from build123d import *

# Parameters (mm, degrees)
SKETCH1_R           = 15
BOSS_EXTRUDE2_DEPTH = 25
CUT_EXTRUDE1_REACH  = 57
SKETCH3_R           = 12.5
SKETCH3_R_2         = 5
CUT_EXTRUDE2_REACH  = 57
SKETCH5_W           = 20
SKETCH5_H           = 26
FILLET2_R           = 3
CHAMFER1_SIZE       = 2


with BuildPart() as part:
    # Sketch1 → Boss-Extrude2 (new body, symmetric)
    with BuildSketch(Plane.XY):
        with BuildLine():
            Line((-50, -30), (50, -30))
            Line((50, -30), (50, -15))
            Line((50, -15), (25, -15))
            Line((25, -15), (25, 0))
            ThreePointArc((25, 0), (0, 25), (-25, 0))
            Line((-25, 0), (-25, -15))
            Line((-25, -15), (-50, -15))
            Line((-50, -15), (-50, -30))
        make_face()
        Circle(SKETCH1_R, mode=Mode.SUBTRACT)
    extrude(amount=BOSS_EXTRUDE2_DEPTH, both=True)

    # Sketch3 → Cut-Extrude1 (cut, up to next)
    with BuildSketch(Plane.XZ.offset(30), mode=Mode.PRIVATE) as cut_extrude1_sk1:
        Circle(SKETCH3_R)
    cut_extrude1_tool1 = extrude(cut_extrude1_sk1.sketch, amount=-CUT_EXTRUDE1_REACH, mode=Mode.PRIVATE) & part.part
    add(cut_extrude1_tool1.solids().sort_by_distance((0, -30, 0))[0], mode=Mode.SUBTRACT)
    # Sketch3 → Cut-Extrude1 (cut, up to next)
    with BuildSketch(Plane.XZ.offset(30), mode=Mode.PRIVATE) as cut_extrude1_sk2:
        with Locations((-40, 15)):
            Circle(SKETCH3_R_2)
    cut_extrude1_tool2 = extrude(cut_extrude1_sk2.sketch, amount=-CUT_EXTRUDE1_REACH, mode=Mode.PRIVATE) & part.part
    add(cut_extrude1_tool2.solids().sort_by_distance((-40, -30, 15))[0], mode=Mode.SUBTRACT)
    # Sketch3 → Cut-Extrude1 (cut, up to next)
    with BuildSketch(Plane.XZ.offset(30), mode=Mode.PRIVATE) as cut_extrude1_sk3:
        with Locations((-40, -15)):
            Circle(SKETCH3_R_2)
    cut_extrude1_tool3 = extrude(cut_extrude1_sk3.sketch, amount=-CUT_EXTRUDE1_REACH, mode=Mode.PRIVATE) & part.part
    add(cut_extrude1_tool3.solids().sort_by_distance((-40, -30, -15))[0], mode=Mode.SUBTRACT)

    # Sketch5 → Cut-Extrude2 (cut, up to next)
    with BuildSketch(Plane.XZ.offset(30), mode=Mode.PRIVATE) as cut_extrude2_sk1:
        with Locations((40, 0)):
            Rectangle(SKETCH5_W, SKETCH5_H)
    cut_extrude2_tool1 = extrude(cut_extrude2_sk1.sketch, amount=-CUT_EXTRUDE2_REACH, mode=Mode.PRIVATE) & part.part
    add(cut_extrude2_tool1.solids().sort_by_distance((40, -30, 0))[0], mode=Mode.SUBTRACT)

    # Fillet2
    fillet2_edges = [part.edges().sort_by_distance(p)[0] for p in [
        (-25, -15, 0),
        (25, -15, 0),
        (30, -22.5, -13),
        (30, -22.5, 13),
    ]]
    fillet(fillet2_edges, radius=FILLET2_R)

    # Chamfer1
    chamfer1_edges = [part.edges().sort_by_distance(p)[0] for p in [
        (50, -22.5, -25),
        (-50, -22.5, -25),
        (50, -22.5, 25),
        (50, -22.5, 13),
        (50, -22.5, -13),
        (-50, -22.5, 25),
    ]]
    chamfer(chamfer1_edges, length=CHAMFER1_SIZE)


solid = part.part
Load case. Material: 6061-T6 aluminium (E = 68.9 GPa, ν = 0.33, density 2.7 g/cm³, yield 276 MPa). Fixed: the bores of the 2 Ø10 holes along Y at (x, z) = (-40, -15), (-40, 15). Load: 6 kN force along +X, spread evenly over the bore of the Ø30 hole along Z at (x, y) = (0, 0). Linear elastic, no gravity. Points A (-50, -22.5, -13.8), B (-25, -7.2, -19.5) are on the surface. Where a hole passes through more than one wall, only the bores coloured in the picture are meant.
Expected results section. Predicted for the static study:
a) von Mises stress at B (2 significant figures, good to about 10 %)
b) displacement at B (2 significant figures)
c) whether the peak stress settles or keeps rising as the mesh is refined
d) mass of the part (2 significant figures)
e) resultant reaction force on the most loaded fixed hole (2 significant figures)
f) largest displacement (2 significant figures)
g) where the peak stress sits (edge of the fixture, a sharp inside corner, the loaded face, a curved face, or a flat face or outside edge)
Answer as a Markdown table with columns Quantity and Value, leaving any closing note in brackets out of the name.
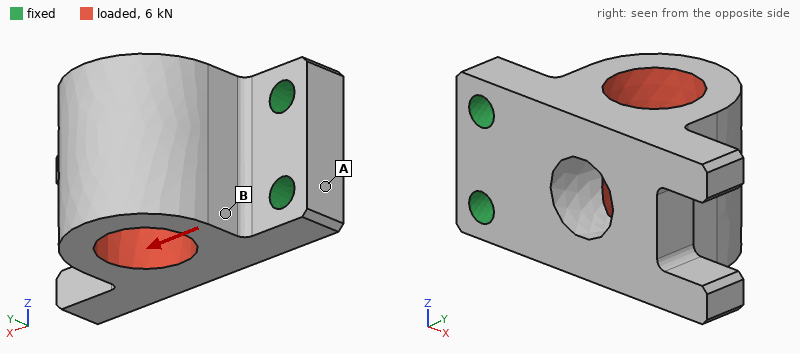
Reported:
| Quantity | Value |
|---|---|
| von Mises stress at B | 30 MPa |
| displacement at B | 0.045 mm |
| whether the peak stress settles or keeps rising as the mesh is refined | keeps rising |
| mass of the part | 290 g |
| resultant reaction force on the most loaded fixed hole | 3.1 kN |
| largest displacement | 0.28 mm |
| where the peak stress sits | edge of the fixture |
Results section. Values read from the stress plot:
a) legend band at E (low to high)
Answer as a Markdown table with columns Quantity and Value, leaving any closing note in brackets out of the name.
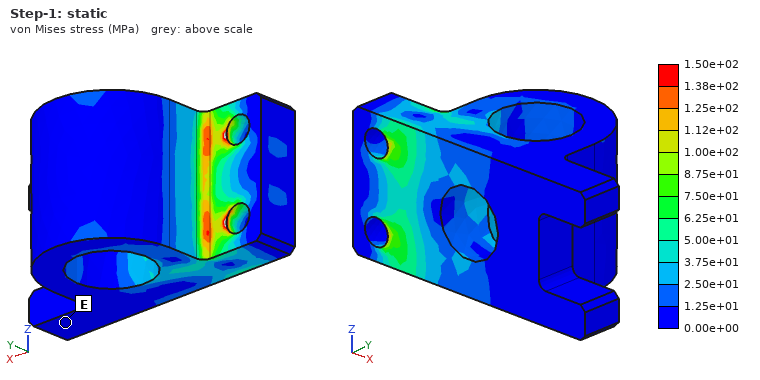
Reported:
| Quantity | Value |
|---|---|
| legend band at E | 0.00e+00 to 1.25e+01 MPa |
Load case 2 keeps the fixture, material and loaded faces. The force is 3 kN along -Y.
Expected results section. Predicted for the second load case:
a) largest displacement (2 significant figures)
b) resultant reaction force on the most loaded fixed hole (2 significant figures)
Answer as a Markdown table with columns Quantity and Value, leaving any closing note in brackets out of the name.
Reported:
| Quantity | Value |
|---|---|
| largest displacement | 0.17 mm |
| resultant reaction force on the most loaded fixed hole | 1.5 kN |
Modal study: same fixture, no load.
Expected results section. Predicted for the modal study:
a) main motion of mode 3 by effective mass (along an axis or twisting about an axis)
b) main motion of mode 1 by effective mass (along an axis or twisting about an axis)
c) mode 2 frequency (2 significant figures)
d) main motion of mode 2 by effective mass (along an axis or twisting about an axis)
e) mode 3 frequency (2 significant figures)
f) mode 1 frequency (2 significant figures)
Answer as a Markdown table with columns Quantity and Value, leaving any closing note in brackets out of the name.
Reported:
| Quantity | Value |
|---|---|
| main motion of mode 3 by effective mass | twisting about X |
| main motion of mode 1 by effective mass | along Y |
| mode 2 frequency | 3400 Hz |
| main motion of mode 2 by effective mass | along Z |
| mode 3 frequency | 4400 Hz |
| mode 1 frequency | 1500 Hz |
